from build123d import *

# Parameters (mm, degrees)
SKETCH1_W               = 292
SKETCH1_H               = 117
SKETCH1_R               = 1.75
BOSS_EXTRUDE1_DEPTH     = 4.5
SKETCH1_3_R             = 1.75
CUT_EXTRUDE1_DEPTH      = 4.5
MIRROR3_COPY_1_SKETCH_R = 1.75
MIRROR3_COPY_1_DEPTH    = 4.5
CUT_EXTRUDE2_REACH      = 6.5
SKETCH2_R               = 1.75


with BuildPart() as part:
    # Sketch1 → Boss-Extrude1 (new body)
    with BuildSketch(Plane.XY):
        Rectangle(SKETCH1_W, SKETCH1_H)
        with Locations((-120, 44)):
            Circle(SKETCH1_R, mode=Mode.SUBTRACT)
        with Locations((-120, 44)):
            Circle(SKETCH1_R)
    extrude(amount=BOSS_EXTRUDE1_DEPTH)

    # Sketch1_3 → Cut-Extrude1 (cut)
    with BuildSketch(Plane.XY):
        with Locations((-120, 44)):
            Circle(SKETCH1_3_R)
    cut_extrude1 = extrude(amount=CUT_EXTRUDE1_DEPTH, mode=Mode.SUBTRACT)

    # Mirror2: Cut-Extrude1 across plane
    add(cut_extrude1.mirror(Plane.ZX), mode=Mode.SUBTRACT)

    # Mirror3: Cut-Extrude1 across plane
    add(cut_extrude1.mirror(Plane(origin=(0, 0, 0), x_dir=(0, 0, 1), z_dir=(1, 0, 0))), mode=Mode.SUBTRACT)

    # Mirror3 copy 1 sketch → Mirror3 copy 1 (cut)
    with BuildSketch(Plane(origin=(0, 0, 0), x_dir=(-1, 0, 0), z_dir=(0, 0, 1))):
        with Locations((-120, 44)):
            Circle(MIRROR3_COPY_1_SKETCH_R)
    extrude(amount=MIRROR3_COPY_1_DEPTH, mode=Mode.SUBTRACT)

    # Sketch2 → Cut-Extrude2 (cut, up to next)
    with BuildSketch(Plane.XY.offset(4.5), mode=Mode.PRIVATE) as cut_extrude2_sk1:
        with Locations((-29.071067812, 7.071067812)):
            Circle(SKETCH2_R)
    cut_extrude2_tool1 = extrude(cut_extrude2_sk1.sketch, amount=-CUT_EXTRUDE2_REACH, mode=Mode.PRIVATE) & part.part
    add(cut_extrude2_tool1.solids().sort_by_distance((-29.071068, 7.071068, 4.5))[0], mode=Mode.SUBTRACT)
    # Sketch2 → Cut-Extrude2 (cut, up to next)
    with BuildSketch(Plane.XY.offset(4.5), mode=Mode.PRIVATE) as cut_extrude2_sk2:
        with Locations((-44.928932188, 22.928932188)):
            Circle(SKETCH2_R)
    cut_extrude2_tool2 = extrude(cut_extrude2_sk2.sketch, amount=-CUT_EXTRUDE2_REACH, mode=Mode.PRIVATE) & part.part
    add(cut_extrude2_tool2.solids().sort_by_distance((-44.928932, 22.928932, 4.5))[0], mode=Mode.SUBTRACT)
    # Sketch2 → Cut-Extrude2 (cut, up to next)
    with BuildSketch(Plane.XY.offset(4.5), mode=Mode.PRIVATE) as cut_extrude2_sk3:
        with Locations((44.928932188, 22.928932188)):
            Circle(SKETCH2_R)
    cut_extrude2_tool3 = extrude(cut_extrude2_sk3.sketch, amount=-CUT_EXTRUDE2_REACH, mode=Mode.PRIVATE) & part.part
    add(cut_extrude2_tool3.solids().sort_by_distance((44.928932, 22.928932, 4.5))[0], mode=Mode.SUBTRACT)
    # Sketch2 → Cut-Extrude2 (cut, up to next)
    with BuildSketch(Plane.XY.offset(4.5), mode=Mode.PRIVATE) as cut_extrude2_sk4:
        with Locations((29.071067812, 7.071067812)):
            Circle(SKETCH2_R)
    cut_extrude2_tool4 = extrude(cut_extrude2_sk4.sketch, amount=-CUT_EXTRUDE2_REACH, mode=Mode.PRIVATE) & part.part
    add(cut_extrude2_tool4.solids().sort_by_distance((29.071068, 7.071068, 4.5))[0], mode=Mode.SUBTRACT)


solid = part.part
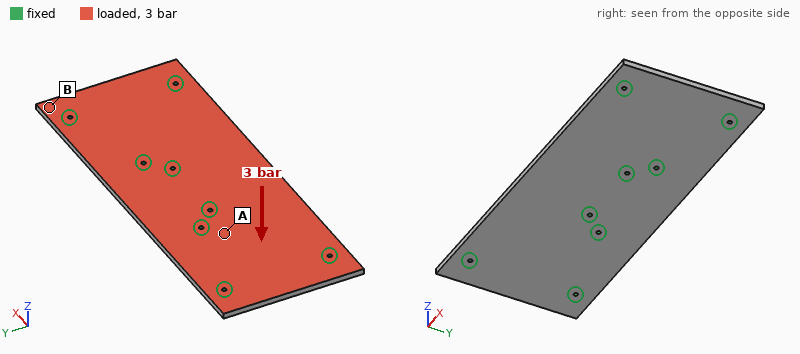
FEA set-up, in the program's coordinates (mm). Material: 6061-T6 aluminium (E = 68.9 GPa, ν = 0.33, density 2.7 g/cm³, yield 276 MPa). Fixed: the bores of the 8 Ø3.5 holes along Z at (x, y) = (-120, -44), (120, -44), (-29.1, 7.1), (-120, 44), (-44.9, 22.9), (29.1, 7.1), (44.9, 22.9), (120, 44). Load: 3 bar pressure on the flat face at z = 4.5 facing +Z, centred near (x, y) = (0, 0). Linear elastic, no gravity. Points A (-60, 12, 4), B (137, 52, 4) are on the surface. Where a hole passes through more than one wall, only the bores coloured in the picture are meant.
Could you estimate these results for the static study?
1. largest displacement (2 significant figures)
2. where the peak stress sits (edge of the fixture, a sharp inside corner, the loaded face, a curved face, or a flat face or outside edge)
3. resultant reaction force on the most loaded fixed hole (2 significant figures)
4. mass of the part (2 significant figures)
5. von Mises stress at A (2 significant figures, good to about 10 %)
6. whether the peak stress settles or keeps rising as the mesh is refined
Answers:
1.1 mm
edge of the fixture
1.8 kN
410 g
42 MPa
keeps rising
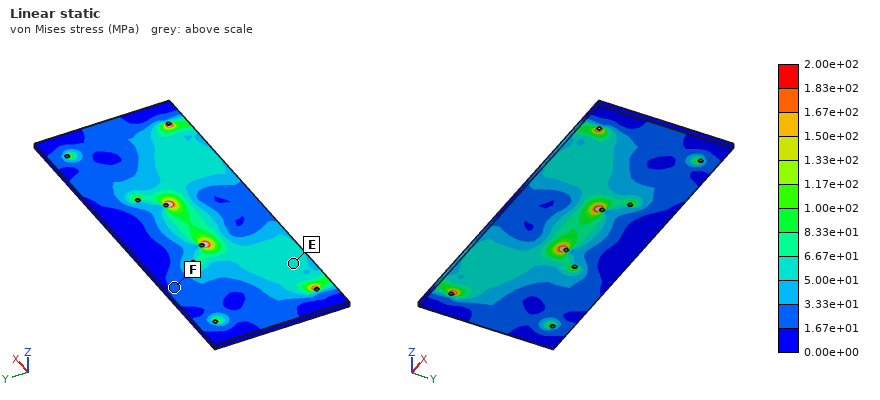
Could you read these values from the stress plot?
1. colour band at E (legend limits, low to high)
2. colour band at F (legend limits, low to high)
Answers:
5.00e+01 to 6.67e+01 MPa
1.67e+01 to 3.33e+01 MPa
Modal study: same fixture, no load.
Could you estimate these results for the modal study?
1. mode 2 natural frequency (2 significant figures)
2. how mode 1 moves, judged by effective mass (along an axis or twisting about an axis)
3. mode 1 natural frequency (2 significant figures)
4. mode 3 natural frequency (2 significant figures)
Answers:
1500 Hz
along Z
990 Hz
2000 Hz
